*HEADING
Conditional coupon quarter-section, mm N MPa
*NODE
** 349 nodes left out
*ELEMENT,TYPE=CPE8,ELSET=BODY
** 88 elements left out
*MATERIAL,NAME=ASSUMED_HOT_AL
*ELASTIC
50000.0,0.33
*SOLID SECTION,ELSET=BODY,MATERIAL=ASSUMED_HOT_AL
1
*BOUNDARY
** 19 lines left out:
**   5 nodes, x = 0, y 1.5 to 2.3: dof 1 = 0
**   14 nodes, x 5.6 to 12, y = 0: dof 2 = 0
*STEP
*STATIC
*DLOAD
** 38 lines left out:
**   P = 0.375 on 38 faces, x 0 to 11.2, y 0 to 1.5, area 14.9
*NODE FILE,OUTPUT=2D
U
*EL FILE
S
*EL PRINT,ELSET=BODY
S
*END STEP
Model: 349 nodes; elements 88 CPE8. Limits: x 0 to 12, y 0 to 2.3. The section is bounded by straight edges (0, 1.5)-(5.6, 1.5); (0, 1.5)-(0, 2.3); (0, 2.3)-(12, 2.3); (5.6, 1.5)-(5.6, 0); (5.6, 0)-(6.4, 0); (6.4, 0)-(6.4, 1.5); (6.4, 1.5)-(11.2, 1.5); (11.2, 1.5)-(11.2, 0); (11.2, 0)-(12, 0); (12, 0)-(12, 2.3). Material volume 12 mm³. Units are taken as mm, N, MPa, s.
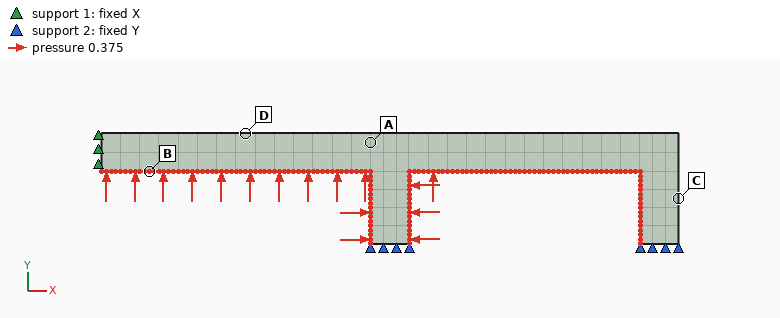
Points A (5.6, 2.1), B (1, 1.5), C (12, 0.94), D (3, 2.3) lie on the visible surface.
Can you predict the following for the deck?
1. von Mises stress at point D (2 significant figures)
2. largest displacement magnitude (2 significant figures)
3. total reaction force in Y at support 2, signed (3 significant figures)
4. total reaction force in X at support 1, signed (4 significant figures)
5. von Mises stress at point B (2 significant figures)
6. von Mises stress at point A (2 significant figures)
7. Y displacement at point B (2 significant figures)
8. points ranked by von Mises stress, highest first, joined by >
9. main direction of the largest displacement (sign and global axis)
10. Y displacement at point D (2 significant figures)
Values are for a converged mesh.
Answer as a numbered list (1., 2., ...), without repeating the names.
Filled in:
1. 8.1 MPa
2. 0.011 mm
3. -3.90 N
4. -0.5625 N
5. 19 MPa
6. 13 MPa
7. 0.011 mm
8. B > A > D > C
9. +Y
10. 0.0069 mm
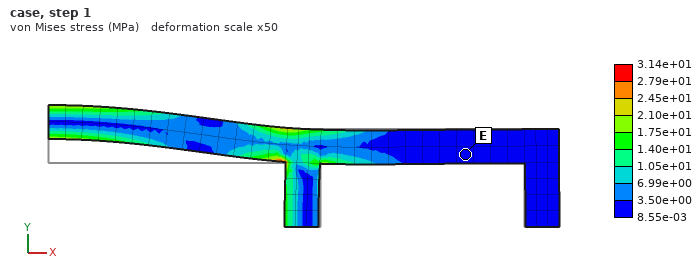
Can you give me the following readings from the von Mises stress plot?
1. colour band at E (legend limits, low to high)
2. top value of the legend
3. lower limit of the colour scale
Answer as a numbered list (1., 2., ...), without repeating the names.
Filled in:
1. 8.55e-03 to 3.50e+00 MPa
2. 3.14e+01 MPa
3. 8.55e-03 MPa
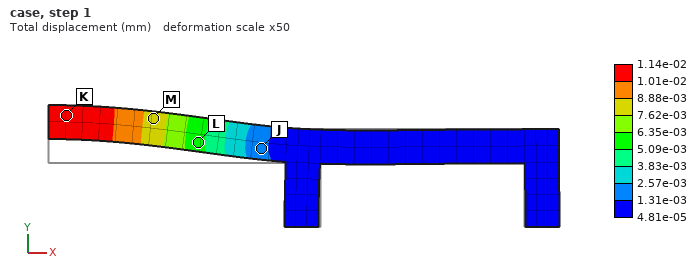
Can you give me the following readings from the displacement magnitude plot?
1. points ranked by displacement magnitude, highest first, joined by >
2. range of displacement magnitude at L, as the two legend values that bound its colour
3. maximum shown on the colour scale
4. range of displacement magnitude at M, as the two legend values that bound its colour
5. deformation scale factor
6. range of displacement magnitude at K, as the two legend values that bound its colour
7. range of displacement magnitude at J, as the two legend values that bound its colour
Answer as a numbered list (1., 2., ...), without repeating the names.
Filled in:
1. K > M > L > J
2. 5.09e-03 to 6.35e-03 mm
3. 1.14e-02 mm
4. 7.62e-03 to 8.88e-03 mm
5. 50
6. 1.01e-02 to 1.14e-02 mm
7. 1.31e-03 to 2.57e-03 mm
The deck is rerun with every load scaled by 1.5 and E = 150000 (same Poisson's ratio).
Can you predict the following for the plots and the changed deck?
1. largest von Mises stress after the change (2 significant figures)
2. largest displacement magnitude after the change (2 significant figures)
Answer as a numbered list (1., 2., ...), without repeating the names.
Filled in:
1. 47 MPa
2. 0.0057 mm
